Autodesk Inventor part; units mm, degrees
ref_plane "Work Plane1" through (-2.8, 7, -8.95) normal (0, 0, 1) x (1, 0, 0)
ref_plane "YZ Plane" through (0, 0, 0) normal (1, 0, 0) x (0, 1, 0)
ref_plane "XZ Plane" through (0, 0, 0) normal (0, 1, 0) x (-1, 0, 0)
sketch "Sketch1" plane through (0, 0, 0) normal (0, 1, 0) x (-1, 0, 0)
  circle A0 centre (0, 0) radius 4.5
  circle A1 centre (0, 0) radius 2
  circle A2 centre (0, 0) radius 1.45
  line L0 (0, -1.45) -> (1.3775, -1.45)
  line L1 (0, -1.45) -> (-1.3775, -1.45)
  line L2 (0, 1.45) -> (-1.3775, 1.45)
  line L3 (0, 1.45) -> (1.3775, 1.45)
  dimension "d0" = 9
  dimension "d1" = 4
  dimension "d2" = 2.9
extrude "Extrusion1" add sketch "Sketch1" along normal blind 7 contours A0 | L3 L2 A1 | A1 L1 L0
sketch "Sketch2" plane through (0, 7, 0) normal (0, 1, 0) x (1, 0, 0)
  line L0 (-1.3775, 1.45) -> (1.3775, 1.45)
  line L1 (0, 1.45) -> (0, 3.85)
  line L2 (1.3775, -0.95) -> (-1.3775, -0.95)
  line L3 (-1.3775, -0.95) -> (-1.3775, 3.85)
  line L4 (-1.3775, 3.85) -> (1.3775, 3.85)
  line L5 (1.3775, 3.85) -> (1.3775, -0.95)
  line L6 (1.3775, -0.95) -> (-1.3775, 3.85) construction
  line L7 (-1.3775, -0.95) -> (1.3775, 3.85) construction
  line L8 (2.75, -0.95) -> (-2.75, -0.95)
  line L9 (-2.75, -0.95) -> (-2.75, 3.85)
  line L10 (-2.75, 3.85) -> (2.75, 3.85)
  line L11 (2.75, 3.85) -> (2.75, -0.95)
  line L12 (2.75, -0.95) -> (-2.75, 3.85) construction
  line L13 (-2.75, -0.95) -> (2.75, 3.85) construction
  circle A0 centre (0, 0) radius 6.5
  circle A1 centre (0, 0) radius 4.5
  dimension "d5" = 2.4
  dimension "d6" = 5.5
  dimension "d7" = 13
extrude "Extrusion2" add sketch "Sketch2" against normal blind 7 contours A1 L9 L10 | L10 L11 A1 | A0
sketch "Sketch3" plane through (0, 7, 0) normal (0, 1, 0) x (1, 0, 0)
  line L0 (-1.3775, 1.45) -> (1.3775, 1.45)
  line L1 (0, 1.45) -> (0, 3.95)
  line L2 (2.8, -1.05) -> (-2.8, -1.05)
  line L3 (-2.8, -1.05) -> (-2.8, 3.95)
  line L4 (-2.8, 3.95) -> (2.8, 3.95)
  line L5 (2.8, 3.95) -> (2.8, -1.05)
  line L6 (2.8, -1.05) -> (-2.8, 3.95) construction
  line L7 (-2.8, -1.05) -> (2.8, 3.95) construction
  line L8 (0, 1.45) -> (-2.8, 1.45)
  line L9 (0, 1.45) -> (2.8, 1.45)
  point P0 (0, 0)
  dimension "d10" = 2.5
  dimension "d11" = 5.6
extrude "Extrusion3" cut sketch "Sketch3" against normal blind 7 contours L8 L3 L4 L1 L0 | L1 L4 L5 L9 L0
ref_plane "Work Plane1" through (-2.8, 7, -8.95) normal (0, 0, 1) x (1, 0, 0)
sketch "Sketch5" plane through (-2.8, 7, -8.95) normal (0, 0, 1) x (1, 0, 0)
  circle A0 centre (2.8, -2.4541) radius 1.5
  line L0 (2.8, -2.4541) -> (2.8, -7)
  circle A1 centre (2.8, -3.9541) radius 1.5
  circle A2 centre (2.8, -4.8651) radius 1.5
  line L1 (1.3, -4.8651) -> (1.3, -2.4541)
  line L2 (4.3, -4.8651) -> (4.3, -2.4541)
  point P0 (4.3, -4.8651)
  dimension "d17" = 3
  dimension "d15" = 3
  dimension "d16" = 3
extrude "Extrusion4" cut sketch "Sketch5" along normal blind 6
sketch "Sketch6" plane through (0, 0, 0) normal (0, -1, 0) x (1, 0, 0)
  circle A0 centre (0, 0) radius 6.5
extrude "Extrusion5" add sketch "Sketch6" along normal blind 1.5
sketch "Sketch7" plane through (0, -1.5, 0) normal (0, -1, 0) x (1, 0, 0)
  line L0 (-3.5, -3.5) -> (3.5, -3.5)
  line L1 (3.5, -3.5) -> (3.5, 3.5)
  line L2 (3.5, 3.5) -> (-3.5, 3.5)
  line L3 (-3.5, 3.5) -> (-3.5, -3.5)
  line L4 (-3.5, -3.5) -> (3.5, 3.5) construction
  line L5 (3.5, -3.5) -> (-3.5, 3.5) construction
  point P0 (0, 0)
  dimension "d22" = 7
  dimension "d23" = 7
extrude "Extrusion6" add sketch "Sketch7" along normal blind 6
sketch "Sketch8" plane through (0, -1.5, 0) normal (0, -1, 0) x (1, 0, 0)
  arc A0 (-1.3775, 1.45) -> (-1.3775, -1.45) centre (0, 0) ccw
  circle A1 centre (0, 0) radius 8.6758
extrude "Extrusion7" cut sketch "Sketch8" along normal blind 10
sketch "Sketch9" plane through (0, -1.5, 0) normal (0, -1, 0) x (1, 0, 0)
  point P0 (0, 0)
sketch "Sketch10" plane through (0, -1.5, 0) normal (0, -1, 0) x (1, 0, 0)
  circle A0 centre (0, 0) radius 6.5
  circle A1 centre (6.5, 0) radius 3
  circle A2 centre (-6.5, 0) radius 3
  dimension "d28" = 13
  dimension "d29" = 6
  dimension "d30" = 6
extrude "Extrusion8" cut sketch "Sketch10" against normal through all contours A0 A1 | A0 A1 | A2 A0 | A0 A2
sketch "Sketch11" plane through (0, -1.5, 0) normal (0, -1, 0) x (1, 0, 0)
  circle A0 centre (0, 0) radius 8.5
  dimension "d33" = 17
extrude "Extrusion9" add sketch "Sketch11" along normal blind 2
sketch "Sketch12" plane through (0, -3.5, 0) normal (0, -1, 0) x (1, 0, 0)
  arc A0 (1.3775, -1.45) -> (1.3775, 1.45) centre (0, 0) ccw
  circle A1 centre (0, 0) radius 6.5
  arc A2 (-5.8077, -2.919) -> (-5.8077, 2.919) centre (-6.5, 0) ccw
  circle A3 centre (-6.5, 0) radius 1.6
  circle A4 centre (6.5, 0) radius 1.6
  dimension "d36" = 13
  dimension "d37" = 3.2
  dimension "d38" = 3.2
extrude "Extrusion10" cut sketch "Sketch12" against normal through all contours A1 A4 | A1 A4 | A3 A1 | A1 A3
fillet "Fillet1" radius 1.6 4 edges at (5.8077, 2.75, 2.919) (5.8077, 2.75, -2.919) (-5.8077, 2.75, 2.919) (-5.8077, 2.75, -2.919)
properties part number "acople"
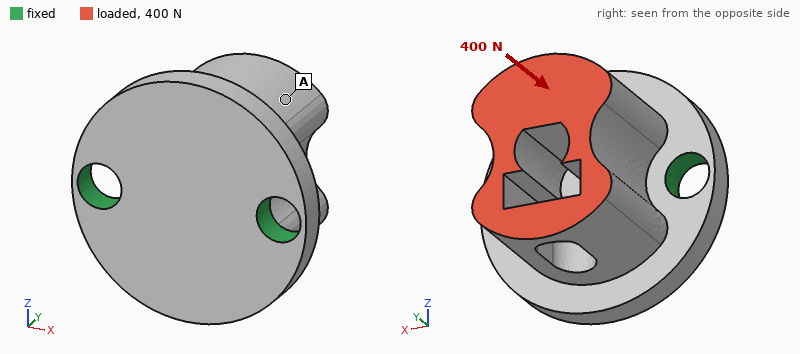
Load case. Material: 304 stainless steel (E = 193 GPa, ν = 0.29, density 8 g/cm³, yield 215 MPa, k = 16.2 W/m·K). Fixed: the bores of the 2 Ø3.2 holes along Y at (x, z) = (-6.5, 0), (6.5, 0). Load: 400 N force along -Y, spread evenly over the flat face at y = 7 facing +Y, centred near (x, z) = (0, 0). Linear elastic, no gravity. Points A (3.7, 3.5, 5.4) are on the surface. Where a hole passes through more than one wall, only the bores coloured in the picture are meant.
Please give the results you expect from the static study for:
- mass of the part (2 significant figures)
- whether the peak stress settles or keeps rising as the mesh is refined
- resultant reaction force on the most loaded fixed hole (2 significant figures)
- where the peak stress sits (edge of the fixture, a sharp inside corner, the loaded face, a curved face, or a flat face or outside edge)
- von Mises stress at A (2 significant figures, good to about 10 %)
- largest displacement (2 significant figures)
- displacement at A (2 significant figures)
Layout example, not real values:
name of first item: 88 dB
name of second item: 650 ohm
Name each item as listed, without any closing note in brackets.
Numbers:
mass of the part: 8.8 g
whether the peak stress settles or keeps rising as the mesh is refined: keeps rising
resultant reaction force on the most loaded fixed hole: 210 N
where the peak stress sits: edge of the fixture
von Mises stress at A: 5.1 MPa
largest displacement: 1.6 µm
displacement at A: 1.3 µm
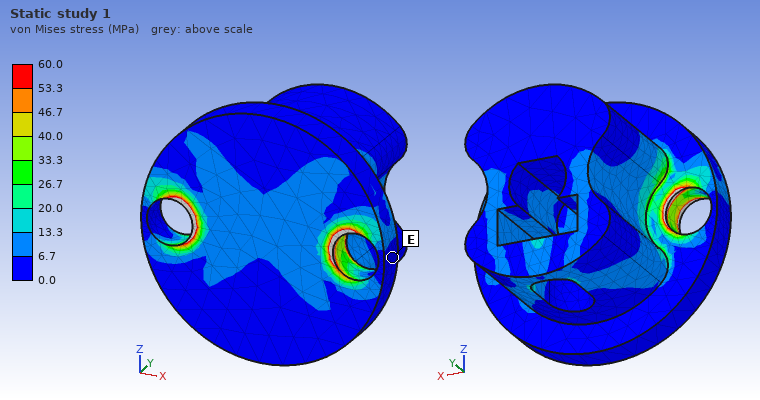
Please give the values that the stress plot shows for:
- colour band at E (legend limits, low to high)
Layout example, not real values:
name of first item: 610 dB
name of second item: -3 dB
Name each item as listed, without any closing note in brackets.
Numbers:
colour band at E: 0.0 to 6.7 MPa
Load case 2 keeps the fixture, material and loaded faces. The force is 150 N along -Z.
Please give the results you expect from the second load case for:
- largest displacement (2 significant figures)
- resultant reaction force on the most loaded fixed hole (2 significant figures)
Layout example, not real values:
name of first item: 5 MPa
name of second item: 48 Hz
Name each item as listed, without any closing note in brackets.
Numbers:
largest displacement: 7.1 µm
resultant reaction force on the most loaded fixed hole: 75 N
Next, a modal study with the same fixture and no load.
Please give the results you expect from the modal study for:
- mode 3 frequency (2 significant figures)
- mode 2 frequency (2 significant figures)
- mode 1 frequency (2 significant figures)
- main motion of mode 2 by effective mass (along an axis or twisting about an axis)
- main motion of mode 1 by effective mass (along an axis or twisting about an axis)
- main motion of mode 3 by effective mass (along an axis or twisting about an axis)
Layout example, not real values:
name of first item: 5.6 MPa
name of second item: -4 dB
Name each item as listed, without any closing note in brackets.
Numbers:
mode 3 frequency: 39 kHz
mode 2 frequency: 32 kHz
mode 1 frequency: 15 kHz
main motion of mode 2 by effective mass: along X
main motion of mode 1 by effective mass: along Z
main motion of mode 3 by effective mass: along Y
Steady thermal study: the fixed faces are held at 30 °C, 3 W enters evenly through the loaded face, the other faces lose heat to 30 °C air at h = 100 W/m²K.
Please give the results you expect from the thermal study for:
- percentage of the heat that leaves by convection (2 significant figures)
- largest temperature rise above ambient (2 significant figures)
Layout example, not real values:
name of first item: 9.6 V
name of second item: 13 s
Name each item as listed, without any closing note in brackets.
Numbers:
percentage of the heat that leaves by convection: 38 %
largest temperature rise above ambient: 30 K
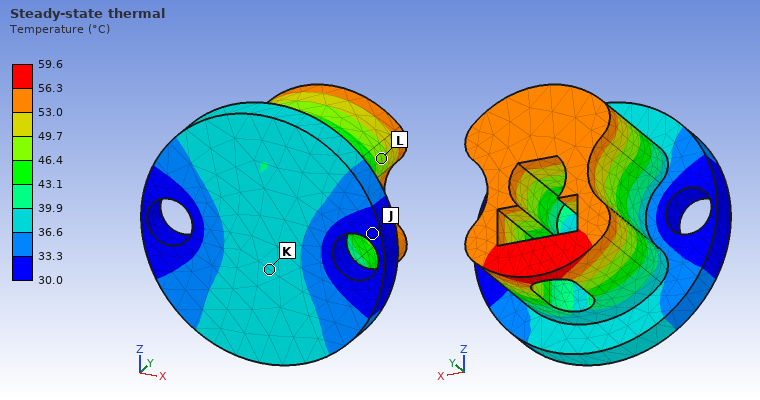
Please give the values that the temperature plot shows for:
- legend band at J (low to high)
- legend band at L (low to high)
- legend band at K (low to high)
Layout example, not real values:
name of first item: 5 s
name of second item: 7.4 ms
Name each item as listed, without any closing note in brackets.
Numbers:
legend band at J: 30.0 to 33.3 °C
legend band at L: 46.4 to 49.7 °C
legend band at K: 36.6 to 39.9 °C
